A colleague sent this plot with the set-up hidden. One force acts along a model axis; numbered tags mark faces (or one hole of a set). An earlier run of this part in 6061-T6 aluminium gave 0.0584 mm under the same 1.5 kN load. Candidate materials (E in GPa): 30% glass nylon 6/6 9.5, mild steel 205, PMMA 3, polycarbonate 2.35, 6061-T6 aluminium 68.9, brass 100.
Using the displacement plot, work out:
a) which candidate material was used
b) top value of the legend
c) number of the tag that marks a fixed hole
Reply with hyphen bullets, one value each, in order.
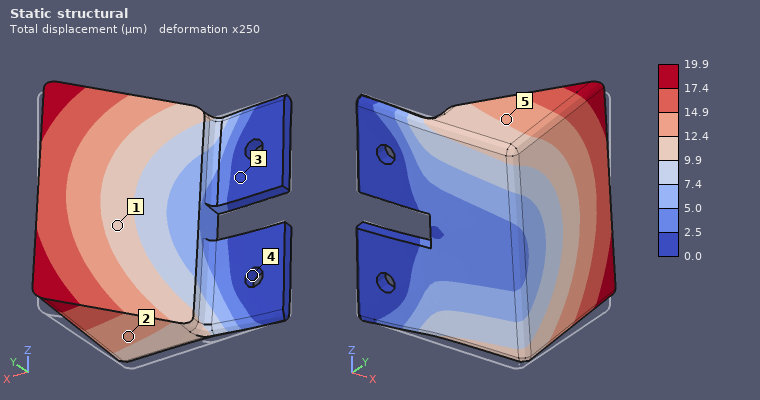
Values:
- mild steel
- 19.9 µm
- 4
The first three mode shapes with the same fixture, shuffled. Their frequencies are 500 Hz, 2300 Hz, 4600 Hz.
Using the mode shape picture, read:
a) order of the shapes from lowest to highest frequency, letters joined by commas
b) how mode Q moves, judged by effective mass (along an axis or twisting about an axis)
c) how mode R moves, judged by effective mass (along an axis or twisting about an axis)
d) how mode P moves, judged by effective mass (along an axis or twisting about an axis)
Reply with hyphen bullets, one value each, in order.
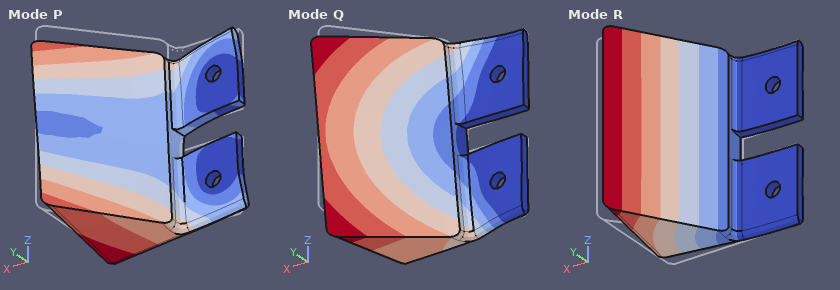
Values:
- R, Q, P
- along Z
- along Y
- along Z
